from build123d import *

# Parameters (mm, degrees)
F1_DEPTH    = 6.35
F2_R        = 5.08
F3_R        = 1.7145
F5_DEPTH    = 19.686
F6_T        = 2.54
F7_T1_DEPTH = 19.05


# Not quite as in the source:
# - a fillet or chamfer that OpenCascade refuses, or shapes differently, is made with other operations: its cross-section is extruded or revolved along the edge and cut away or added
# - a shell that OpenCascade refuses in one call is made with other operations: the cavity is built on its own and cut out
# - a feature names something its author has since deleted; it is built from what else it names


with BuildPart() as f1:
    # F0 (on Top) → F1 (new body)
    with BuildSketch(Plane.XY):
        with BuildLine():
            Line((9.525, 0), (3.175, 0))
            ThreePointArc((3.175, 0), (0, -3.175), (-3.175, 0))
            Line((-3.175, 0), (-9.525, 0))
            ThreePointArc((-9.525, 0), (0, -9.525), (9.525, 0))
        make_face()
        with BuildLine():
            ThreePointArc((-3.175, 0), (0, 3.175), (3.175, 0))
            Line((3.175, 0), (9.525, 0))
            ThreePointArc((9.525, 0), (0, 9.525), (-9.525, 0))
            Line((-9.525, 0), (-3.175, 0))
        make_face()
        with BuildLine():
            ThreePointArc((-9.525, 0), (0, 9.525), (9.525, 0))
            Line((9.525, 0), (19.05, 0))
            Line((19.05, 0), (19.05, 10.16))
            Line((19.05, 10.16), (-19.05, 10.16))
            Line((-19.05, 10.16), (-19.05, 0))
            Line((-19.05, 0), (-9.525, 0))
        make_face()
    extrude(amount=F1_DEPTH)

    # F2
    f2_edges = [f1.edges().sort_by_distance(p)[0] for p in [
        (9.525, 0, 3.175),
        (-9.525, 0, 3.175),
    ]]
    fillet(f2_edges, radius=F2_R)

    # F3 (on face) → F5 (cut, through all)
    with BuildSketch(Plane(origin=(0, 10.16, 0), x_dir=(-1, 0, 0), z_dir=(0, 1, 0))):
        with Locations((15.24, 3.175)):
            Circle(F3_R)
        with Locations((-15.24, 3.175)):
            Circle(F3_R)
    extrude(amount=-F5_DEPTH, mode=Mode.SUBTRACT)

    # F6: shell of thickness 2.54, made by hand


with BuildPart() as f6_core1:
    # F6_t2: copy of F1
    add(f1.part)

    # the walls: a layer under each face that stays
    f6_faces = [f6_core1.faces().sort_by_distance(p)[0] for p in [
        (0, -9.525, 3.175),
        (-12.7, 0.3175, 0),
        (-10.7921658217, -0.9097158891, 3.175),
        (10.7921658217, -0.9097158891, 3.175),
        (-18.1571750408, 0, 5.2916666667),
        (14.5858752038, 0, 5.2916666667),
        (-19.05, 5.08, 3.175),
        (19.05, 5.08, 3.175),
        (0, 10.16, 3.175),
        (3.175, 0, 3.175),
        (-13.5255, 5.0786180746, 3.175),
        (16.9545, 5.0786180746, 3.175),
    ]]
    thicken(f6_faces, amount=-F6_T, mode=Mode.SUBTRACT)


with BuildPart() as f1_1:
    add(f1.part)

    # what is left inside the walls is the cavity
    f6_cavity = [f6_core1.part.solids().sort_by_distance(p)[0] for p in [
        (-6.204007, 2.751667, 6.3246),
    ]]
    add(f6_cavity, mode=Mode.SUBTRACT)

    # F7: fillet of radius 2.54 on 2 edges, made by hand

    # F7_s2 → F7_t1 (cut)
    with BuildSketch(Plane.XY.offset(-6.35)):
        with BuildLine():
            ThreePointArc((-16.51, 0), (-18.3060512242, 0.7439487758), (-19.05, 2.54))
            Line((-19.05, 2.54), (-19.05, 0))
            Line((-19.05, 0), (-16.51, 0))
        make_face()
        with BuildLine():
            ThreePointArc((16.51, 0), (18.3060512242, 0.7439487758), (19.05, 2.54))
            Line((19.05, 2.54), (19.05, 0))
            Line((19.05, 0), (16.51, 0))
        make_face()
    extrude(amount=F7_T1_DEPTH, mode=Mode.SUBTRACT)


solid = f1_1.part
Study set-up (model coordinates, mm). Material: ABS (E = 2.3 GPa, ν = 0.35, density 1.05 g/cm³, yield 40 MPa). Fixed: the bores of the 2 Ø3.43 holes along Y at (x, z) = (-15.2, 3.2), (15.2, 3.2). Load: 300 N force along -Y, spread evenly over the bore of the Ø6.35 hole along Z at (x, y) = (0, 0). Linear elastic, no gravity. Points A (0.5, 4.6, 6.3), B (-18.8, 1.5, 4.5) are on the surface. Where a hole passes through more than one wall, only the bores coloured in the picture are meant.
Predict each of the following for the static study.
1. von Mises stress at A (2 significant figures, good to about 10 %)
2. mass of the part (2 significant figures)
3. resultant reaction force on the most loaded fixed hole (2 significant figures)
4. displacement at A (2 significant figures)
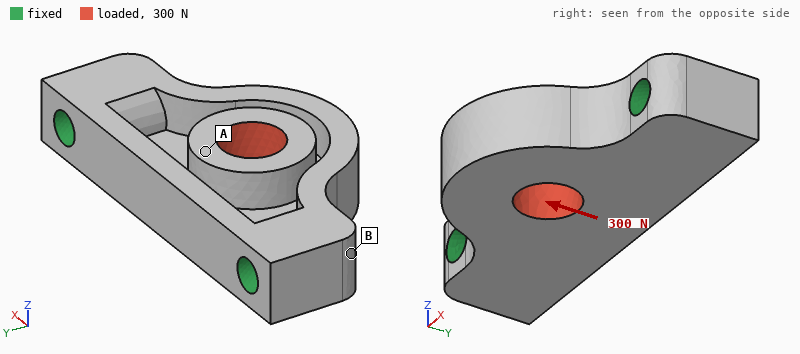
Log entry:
4.5 MPa
2.6 g
160 N
0.12 mm
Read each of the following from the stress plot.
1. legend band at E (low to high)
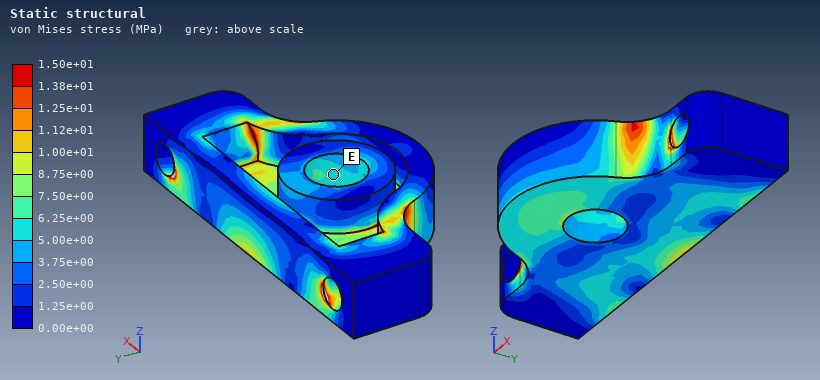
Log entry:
5.00e+00 to 6.25e+00 MPa
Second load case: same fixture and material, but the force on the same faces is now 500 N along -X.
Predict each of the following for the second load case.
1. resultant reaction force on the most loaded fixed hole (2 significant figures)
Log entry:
260 N
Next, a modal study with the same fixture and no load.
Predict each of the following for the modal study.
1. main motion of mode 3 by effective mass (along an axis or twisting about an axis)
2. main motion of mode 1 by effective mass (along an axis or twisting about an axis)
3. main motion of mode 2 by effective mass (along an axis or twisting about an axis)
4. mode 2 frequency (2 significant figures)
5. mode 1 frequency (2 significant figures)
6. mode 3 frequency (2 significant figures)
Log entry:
along Y
along Z
along Z
8100 Hz
4400 Hz
10 kHz
